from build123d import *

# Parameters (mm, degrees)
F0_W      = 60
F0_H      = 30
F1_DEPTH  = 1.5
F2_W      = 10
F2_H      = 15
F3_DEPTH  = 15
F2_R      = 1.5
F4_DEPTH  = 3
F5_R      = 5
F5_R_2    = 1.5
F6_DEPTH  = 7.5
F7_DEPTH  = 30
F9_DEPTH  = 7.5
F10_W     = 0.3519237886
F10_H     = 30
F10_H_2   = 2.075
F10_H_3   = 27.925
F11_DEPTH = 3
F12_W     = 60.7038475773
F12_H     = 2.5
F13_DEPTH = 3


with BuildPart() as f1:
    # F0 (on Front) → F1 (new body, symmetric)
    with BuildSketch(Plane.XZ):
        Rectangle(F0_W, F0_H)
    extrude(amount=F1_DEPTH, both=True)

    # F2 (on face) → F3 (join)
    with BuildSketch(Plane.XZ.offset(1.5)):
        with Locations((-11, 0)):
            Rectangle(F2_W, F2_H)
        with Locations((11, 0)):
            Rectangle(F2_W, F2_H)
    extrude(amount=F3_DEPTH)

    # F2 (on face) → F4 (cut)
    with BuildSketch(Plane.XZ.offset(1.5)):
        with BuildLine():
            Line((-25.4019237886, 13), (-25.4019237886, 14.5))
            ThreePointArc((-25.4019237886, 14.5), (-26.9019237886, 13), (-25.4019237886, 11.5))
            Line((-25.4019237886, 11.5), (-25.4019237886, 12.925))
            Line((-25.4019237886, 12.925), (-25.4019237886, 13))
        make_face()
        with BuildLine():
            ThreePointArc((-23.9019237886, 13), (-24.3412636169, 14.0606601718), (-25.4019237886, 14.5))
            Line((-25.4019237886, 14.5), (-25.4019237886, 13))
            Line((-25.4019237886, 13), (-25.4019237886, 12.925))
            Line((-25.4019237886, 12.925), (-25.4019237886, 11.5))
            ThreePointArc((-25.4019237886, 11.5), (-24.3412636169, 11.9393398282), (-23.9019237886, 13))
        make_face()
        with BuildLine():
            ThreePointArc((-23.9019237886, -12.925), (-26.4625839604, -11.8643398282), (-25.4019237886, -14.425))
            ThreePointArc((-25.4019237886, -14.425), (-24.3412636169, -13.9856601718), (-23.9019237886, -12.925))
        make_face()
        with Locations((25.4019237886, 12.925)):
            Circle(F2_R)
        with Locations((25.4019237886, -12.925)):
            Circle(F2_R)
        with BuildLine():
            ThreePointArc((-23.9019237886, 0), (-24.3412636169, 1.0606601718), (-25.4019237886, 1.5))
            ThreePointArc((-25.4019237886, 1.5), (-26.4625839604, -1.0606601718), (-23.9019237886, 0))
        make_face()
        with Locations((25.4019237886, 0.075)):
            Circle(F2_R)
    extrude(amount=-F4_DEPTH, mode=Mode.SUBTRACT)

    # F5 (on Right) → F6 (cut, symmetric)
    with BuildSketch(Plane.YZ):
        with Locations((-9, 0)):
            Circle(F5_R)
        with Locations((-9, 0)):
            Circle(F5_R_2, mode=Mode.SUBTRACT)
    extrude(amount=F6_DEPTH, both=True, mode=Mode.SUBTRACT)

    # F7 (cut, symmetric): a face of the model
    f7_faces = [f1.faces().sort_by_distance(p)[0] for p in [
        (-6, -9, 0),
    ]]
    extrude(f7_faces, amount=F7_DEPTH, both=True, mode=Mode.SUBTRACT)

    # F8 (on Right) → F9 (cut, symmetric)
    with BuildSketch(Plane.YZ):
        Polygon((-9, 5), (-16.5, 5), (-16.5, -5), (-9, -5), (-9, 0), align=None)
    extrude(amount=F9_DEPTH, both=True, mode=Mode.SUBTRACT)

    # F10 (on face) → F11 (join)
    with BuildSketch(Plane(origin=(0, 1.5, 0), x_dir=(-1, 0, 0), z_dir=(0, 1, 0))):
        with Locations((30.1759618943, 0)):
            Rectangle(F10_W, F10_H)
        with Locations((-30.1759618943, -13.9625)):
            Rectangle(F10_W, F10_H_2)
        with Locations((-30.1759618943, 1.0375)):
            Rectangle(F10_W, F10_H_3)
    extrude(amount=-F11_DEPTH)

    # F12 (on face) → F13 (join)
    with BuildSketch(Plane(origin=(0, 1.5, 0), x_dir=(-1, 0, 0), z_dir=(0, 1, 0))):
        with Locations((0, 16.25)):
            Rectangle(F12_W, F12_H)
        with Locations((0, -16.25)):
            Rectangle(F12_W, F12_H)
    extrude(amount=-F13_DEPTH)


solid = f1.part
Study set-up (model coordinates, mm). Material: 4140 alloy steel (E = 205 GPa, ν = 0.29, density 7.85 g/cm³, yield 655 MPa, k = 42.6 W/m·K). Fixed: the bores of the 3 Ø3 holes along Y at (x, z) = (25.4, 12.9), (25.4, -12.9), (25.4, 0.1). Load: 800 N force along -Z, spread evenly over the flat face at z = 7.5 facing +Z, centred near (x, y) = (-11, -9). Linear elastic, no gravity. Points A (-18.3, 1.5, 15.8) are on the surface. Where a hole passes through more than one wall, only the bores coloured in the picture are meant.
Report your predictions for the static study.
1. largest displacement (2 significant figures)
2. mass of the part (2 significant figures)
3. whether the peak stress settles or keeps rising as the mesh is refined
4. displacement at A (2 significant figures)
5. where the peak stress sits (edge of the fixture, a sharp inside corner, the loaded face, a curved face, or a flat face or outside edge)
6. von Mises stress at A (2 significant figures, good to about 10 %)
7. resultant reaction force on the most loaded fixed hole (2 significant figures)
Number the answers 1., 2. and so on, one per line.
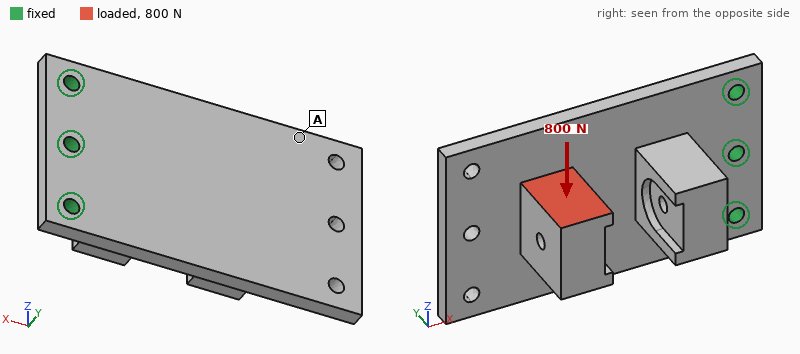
1. 85 µm
2. 81 g
3. keeps rising
4. 67 µm
5. edge of the fixture
6. 19 MPa
7. 1.1 kN
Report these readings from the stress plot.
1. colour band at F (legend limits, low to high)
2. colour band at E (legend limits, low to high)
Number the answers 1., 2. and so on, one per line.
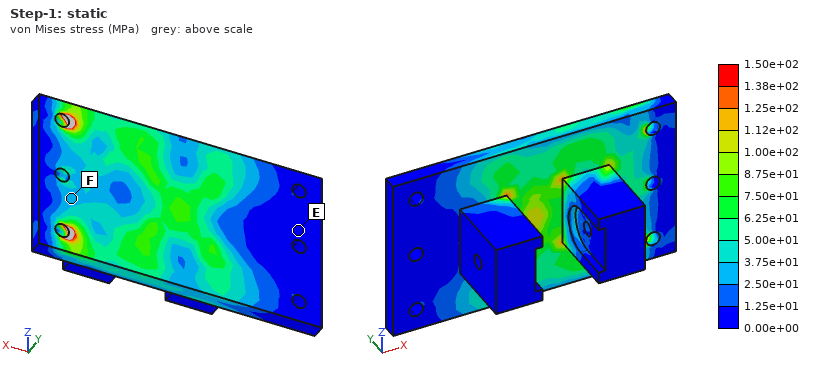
1. 2.50e+01 to 3.75e+01 MPa
2. 0.00e+00 to 1.25e+01 MPa
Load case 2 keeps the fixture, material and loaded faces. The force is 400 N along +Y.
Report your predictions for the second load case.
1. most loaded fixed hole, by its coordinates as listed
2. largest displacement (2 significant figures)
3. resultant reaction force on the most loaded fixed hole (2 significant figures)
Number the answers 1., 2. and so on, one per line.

1. (25.4, 12.9)
2. 0.62 mm
3. 250 N
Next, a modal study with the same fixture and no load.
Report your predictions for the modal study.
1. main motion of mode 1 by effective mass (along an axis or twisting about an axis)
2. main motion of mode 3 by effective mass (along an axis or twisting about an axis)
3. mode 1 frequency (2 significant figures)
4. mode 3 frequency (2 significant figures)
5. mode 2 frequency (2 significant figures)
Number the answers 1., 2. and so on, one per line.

1. along Y
2. along Y
3. 720 Hz
4. 3800 Hz
5. 3000 Hz
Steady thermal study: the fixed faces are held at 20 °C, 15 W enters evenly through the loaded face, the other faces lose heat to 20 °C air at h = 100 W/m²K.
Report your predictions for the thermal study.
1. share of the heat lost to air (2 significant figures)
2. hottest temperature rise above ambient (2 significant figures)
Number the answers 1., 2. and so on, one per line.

1. 81 %
2. 63 K
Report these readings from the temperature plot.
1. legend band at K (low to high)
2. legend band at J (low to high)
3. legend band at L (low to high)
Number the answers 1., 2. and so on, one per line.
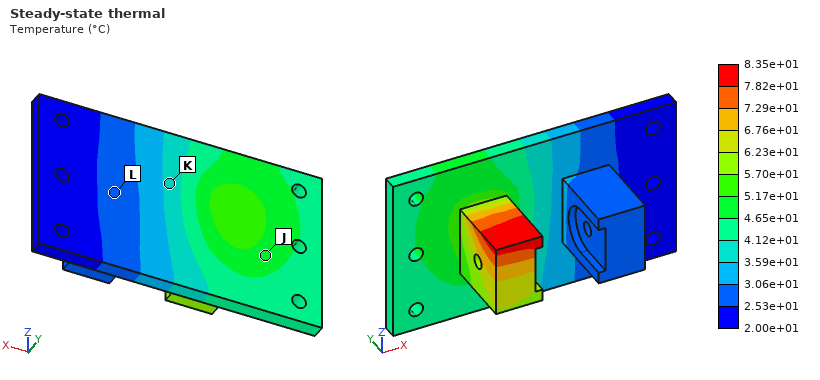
1. 3.59e+01 to 4.12e+01 °C
2. 4.65e+01 to 5.17e+01 °C
3. 2.53e+01 to 3.06e+01 °C
